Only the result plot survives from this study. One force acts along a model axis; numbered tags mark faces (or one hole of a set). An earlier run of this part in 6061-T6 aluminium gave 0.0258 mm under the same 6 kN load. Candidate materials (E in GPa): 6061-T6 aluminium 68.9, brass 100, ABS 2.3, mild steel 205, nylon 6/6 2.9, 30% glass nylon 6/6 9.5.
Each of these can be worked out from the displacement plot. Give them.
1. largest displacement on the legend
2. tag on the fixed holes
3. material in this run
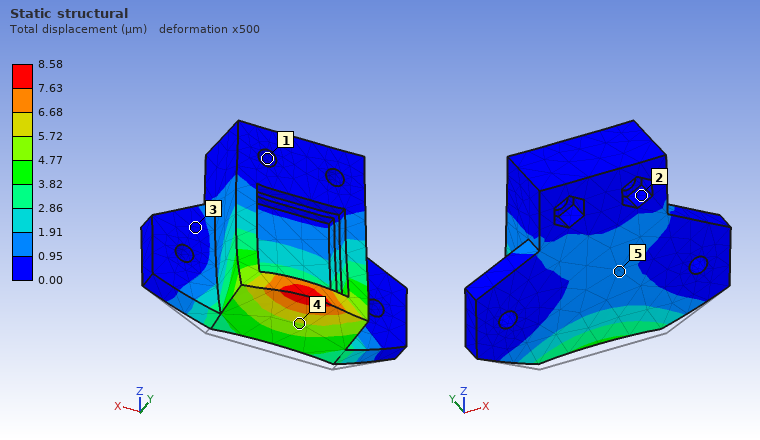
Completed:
8.58 µm
1
mild steel
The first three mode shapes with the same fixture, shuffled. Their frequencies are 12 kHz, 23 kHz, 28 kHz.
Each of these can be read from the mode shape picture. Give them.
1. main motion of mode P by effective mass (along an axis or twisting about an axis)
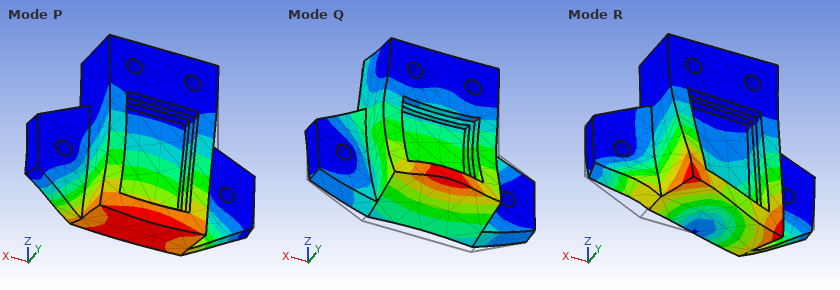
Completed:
along Y
